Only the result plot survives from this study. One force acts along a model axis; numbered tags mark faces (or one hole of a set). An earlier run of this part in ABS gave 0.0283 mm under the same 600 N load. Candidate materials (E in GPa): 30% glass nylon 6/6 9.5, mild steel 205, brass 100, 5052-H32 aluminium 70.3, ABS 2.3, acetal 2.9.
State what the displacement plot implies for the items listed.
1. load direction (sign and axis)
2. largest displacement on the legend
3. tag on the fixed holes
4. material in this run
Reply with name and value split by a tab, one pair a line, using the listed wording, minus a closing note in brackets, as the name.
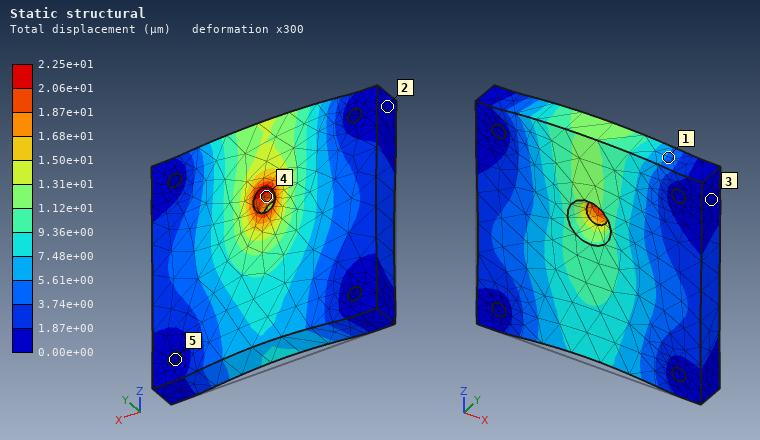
load direction	+Z
largest displacement on the legend	2.25e+01 µm
tag on the fixed holes	5
material in this run	acetal
